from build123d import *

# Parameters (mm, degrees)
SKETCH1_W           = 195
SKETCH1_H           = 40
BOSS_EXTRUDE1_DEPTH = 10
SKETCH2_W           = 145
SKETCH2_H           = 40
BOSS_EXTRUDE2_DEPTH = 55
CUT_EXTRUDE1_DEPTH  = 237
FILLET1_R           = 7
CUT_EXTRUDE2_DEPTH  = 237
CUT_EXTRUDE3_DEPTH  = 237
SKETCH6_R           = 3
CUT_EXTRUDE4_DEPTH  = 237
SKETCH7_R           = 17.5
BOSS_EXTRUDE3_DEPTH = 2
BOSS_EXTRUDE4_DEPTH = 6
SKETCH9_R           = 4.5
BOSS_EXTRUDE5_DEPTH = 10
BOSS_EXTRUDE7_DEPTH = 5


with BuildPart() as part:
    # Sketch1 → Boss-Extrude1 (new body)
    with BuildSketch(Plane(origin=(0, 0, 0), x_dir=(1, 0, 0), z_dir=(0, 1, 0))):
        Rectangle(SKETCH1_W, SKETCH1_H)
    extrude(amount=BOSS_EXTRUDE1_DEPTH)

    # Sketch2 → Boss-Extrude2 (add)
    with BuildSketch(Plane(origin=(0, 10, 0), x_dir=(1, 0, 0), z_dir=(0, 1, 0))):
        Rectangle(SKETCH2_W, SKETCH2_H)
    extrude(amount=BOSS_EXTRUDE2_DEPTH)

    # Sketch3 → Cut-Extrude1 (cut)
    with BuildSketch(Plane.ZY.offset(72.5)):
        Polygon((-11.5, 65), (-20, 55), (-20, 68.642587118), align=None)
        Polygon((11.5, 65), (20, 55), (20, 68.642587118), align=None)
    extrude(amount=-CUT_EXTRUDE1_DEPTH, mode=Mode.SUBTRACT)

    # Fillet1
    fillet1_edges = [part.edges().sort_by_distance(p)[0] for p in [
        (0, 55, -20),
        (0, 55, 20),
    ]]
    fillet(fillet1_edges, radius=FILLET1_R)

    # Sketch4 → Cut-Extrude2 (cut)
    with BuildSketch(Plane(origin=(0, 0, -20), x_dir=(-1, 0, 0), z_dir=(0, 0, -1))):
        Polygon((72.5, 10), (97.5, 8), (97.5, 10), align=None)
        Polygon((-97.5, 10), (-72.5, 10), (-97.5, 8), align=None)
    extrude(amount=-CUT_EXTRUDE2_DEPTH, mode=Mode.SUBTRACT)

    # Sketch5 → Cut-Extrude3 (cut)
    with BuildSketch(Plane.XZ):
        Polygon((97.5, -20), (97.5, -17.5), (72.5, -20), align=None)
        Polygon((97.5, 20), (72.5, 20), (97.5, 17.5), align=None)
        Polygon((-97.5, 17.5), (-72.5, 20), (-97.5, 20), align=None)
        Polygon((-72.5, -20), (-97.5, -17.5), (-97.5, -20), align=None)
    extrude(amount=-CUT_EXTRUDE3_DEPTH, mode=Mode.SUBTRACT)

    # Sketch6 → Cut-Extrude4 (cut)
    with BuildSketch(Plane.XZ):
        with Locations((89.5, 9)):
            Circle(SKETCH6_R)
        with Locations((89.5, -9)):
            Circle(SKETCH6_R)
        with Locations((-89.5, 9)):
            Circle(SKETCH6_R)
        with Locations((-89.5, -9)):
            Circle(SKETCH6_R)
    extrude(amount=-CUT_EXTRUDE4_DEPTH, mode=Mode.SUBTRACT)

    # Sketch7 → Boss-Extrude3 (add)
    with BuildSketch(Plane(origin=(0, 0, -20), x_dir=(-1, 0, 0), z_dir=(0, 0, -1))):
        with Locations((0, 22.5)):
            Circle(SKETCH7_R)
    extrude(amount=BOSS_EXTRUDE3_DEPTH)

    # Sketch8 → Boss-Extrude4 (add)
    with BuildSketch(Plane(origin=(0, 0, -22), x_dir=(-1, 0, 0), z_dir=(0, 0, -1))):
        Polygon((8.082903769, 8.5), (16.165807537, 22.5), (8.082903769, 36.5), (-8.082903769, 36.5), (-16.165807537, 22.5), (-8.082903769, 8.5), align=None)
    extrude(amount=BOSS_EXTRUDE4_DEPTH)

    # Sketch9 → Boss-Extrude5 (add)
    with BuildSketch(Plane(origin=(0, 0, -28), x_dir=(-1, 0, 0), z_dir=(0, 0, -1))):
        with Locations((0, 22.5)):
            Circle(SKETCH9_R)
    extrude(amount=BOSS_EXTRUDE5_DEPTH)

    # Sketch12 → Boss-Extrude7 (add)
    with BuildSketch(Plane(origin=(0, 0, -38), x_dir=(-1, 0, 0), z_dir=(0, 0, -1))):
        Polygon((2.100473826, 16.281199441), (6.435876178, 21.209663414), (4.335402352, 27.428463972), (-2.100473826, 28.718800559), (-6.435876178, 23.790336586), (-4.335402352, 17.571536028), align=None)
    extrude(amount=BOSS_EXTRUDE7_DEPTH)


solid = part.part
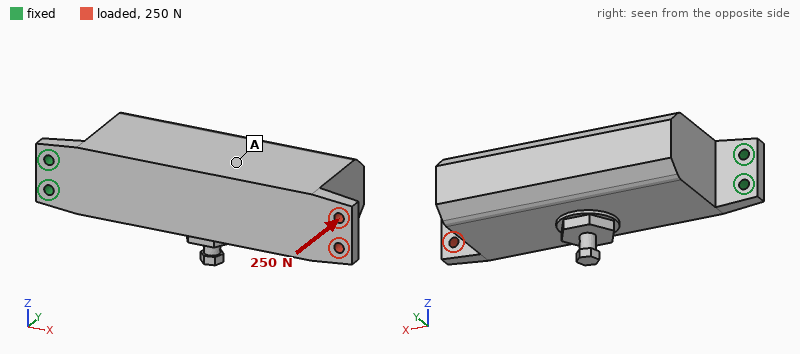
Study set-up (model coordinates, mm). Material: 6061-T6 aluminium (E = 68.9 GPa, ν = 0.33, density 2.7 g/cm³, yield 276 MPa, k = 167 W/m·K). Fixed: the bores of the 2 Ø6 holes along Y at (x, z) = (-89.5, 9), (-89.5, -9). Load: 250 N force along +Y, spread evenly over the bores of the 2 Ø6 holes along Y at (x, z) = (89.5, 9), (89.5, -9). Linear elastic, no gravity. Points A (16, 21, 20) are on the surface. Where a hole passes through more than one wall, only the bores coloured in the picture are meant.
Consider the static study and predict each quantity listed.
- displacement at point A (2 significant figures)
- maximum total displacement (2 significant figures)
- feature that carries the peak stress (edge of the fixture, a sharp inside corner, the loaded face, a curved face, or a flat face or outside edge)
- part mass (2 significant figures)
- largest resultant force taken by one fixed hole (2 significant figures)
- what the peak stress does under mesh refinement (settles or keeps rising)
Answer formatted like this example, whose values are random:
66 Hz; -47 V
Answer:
0.46 mm; 0.85 mm; edge of the fixture; 1.0 kg; 130 N; keeps rising
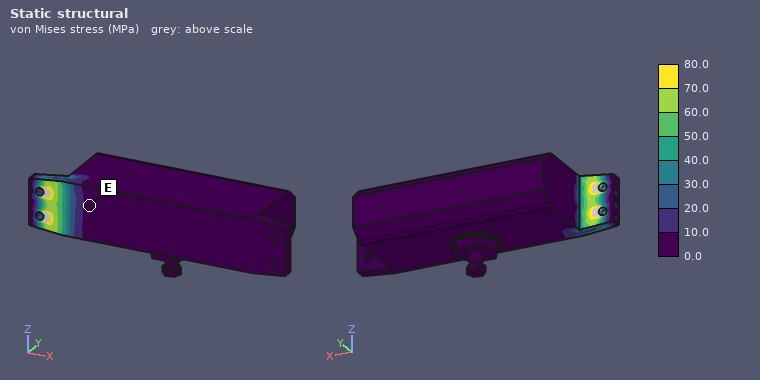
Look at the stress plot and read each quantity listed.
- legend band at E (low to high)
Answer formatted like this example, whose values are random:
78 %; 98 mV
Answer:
0.0 to 10.0 MPa
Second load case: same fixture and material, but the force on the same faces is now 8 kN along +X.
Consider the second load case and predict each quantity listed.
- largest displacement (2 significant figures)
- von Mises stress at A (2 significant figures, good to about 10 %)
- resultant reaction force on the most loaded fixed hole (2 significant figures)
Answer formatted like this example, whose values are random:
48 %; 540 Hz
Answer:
0.19 mm; 5.8 MPa; 4.0 kN
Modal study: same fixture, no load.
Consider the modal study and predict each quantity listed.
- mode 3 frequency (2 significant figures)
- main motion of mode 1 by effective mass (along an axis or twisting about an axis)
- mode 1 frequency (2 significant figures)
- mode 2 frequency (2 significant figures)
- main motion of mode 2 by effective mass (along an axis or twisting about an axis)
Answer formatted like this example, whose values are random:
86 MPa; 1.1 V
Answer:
980 Hz; along Y; 150 Hz; 460 Hz; along Z
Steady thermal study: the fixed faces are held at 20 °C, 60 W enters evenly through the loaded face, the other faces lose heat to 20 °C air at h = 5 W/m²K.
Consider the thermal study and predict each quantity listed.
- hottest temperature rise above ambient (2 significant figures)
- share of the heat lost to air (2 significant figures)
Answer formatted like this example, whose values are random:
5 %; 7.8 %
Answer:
71 K; 10 %
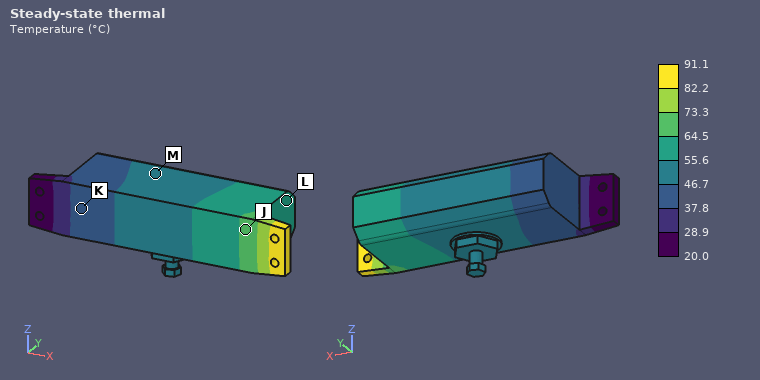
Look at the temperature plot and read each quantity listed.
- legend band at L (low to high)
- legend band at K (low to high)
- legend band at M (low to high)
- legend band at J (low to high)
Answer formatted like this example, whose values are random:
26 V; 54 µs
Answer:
55.6 to 64.5 °C; 37.8 to 46.7 °C; 46.7 to 55.6 °C; 64.5 to 73.3 °C
